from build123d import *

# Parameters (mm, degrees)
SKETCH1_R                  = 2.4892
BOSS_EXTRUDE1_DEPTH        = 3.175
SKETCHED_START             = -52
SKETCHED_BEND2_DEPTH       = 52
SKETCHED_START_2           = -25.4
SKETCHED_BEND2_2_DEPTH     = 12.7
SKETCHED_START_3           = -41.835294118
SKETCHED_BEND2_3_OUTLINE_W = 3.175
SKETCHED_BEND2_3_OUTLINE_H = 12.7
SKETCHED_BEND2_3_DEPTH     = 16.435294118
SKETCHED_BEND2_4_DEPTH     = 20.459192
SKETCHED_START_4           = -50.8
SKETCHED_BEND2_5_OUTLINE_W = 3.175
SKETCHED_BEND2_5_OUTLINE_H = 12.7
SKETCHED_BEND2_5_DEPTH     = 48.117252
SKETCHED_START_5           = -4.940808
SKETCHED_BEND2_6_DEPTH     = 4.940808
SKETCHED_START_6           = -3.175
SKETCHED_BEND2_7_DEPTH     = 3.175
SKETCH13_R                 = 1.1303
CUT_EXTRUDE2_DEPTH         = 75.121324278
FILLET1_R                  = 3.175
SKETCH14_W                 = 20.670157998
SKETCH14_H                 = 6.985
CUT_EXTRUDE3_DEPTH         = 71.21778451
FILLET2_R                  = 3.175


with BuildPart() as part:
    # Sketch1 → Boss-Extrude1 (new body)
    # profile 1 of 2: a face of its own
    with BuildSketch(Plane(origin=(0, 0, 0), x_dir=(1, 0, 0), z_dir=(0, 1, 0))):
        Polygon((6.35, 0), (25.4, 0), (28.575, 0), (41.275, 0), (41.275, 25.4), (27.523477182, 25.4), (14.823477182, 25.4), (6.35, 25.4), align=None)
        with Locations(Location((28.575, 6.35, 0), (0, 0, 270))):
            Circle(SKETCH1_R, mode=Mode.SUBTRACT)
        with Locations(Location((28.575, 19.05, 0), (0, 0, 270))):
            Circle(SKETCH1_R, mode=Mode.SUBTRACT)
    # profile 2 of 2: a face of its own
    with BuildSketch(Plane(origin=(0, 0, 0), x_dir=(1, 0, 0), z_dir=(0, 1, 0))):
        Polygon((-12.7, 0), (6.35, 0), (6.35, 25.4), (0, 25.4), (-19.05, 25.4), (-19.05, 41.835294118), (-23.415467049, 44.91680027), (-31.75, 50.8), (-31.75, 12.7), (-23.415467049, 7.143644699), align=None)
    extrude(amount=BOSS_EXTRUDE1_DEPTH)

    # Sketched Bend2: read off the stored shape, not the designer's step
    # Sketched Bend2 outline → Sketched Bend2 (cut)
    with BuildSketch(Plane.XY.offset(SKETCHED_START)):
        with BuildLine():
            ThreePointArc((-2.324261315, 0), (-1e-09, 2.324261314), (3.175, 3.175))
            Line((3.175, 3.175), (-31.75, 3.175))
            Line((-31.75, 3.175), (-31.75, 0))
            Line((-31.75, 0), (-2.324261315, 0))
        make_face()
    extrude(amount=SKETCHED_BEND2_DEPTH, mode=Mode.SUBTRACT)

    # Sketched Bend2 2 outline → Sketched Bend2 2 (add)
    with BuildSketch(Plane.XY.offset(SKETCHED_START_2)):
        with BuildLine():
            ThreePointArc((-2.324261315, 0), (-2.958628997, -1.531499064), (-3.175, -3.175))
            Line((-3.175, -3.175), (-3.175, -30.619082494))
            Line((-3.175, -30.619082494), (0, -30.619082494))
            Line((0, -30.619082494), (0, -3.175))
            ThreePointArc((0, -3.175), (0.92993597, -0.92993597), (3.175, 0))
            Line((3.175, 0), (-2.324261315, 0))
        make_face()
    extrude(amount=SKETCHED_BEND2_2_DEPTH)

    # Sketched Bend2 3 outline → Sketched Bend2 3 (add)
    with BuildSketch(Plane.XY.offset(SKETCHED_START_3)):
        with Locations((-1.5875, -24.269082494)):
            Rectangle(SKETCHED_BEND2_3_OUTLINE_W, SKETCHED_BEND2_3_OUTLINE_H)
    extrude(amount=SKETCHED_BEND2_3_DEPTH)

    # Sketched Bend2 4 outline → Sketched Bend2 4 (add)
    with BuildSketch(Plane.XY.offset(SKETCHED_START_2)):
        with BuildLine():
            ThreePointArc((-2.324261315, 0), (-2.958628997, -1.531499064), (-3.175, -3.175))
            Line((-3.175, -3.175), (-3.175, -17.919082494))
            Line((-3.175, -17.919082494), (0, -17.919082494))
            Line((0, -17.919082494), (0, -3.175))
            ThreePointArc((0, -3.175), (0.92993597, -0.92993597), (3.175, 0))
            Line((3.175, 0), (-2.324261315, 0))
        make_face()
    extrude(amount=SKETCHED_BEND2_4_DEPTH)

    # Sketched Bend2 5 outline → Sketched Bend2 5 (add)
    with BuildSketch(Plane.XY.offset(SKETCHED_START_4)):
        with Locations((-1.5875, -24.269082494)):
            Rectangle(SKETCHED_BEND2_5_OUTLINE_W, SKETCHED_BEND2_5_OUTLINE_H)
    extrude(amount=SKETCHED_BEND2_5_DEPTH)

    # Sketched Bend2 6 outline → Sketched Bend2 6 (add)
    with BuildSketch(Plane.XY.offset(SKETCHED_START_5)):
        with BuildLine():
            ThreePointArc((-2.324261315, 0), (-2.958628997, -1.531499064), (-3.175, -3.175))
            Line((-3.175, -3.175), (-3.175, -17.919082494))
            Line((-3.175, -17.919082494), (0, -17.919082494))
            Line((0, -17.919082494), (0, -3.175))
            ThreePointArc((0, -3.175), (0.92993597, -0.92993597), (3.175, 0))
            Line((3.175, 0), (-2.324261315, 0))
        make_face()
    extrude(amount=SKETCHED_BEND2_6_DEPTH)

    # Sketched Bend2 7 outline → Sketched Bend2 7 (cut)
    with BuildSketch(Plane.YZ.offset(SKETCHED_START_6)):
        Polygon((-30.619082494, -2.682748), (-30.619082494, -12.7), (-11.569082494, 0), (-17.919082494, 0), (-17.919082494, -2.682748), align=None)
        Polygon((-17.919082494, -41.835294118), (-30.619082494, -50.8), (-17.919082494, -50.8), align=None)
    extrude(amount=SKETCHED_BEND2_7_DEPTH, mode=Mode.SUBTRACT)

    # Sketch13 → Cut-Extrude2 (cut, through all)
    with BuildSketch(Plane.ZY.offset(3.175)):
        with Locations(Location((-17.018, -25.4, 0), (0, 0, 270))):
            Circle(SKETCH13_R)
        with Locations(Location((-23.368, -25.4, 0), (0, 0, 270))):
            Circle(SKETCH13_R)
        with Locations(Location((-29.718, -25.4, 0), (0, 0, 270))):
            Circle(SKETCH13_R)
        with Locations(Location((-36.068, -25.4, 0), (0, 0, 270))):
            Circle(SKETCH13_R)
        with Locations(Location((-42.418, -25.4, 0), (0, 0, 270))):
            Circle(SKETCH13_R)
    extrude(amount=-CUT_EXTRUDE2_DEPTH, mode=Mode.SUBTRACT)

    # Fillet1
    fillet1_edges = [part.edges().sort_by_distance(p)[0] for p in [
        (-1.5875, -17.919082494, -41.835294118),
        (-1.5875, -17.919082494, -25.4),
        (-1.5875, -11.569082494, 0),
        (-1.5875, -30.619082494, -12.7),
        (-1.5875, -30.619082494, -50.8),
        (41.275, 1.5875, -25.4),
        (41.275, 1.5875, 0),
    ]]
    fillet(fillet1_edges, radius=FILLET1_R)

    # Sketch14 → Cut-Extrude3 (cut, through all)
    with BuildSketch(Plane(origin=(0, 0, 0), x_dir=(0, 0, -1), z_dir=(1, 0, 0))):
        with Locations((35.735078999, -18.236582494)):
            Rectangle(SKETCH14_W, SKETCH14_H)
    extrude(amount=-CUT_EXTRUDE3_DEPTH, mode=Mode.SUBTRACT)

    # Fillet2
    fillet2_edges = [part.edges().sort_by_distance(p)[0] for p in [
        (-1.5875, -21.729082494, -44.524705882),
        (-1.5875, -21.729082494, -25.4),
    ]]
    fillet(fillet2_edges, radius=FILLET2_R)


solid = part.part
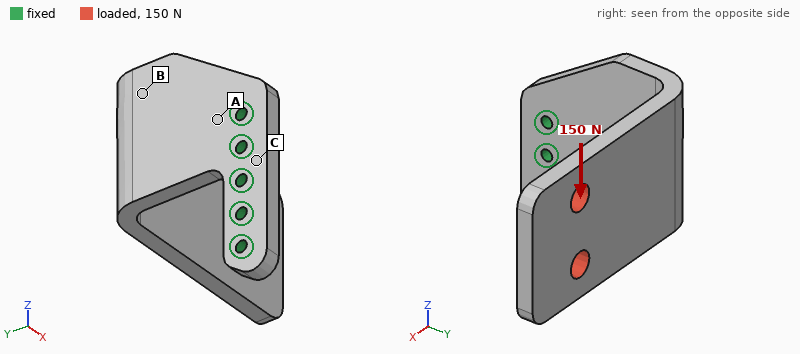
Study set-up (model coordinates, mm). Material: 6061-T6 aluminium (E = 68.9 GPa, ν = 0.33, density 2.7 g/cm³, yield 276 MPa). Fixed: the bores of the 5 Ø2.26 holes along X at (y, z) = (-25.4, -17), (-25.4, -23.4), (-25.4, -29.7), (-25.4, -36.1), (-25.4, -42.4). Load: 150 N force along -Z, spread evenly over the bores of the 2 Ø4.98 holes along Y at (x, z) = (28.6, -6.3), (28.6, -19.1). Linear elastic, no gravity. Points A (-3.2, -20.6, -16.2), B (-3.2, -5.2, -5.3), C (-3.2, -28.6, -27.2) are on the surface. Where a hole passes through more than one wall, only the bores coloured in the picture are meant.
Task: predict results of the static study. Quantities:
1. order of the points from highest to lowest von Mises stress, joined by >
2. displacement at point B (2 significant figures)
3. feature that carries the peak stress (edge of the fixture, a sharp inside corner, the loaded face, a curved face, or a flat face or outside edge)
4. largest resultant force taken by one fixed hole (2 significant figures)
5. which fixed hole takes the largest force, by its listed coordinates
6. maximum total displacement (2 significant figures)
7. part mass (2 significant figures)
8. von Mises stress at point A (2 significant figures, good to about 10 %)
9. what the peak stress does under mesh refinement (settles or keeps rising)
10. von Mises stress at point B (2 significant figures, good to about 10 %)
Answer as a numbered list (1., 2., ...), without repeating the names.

1. A > B > C
2. 0.20 mm
3. edge of the fixture
4. 560 N
5. (-25.4, -17)
6. 0.88 mm
7. 16 g
8. 110 MPa
9. keeps rising
10. 56 MPa
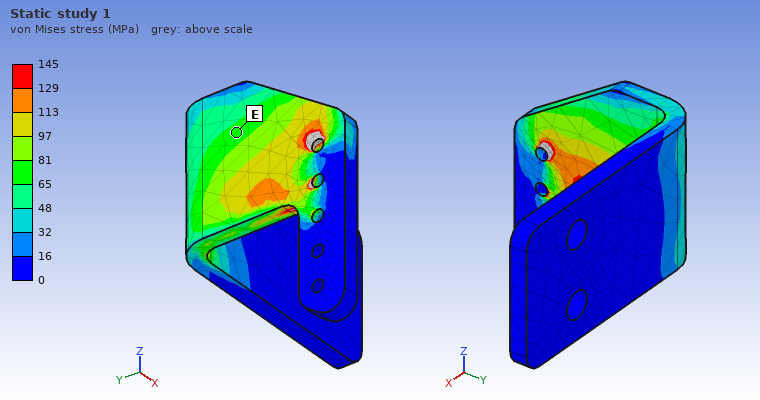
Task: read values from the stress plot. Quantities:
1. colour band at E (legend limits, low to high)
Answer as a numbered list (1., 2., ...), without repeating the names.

1. 65 to 81 MPa
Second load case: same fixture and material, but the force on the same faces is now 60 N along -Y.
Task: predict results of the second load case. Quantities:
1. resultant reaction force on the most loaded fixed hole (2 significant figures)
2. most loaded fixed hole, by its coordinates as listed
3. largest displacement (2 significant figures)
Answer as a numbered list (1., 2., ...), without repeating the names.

1. 79 N
2. (-25.4, -17)
3. 0.70 mm
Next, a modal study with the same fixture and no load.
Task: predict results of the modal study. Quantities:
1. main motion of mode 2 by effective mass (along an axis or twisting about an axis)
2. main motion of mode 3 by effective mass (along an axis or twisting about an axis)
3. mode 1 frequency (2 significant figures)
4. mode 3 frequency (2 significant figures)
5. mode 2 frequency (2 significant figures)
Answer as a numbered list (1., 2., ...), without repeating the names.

1. along Z
2. along X
3. 660 Hz
4. 2100 Hz
5. 1000 Hz
